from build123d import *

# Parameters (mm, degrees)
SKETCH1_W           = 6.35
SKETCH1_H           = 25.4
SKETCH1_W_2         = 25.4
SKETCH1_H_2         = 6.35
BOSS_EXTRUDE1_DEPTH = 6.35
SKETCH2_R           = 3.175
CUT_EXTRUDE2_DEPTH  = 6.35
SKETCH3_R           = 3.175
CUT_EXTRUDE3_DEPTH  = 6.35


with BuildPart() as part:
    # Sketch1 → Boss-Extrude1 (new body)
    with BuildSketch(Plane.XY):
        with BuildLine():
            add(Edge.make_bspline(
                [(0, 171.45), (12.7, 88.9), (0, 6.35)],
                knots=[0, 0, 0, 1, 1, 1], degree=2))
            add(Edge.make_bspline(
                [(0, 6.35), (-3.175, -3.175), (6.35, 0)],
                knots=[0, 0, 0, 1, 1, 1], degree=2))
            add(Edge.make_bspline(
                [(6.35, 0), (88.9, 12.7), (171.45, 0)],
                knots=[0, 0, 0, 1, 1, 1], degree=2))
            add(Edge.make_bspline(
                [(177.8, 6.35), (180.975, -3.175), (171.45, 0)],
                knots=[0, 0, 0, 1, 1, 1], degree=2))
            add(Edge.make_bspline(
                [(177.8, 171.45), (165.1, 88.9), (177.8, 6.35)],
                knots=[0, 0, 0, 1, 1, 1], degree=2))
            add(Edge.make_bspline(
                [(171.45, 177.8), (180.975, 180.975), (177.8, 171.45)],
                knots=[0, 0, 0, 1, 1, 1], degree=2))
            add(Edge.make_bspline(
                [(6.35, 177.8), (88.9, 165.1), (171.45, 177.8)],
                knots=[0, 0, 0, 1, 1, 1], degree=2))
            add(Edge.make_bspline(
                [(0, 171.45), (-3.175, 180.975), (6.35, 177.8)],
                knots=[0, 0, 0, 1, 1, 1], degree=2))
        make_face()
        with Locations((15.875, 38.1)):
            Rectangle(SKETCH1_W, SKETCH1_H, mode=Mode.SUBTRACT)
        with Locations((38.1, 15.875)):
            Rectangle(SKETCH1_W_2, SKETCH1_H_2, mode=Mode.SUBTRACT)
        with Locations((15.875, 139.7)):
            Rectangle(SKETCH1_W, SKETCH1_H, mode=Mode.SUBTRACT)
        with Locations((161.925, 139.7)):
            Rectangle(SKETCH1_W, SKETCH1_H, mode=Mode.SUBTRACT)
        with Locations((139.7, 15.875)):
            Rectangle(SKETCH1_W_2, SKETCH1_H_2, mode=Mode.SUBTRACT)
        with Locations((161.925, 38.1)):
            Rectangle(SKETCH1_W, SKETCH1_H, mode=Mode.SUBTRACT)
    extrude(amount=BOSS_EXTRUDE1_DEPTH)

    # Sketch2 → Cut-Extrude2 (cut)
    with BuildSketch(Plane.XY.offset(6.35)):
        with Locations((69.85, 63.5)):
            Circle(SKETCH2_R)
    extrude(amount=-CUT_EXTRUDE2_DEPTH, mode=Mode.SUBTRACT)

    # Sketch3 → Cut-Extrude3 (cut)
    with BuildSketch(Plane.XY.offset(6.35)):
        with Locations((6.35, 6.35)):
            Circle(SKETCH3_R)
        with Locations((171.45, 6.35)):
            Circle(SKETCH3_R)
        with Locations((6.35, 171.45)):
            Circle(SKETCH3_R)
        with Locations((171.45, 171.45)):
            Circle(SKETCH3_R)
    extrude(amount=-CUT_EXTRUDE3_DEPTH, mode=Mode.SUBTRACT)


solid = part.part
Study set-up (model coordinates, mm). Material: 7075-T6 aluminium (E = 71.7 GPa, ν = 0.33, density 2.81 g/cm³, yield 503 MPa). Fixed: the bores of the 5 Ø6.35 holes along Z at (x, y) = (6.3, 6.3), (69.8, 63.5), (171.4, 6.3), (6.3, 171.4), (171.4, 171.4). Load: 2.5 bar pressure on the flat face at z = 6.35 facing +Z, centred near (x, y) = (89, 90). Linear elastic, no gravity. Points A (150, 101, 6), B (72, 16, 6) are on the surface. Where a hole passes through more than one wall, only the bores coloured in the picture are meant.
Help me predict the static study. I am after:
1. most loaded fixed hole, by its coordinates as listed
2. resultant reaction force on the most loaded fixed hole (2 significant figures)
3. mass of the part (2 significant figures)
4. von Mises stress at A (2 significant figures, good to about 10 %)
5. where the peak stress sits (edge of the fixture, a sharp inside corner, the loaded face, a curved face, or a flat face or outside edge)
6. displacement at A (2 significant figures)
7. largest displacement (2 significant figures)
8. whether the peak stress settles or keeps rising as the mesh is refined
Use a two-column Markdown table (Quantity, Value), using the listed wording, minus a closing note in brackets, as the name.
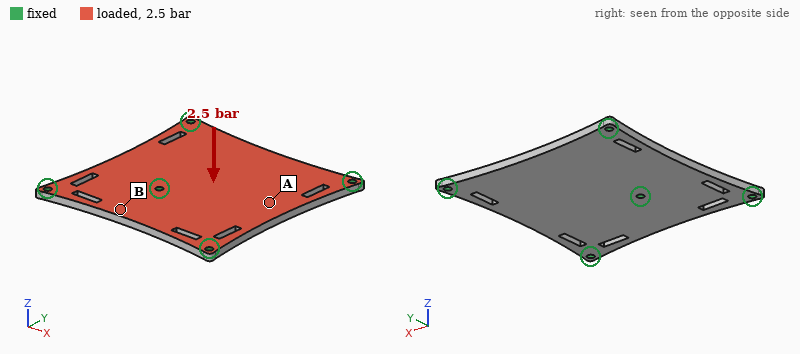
| Quantity | Value |
|---|---|
| most loaded fixed hole, by its coordinates as listed | (69.8, 63.5) |
| resultant reaction force on the most loaded fixed hole | 3.4 kN |
| mass of the part | 490 g |
| von Mises stress at A | 35 MPa |
| where the peak stress sits | edge of the fixture |
| displacement at A | 0.32 mm |
| largest displacement | 0.35 mm |
| whether the peak stress settles or keeps rising as the mesh is refined | keeps rising |
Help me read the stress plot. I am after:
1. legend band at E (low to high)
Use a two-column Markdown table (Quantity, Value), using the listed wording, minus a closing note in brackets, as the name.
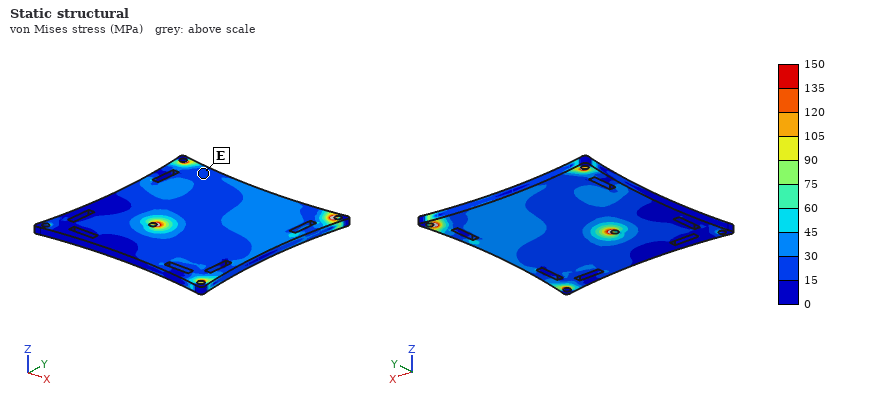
| Quantity | Value |
|---|---|
| legend band at E | 15 to 30 MPa |
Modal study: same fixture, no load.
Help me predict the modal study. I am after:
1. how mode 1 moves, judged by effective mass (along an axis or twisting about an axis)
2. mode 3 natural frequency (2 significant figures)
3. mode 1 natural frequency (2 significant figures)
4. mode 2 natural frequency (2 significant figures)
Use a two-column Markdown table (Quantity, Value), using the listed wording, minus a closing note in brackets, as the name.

| Quantity | Value |
|---|---|
| how mode 1 moves, judged by effective mass | along Z |
| mode 3 natural frequency | 1700 Hz |
| mode 1 natural frequency | 1200 Hz |
| mode 2 natural frequency | 1400 Hz |
